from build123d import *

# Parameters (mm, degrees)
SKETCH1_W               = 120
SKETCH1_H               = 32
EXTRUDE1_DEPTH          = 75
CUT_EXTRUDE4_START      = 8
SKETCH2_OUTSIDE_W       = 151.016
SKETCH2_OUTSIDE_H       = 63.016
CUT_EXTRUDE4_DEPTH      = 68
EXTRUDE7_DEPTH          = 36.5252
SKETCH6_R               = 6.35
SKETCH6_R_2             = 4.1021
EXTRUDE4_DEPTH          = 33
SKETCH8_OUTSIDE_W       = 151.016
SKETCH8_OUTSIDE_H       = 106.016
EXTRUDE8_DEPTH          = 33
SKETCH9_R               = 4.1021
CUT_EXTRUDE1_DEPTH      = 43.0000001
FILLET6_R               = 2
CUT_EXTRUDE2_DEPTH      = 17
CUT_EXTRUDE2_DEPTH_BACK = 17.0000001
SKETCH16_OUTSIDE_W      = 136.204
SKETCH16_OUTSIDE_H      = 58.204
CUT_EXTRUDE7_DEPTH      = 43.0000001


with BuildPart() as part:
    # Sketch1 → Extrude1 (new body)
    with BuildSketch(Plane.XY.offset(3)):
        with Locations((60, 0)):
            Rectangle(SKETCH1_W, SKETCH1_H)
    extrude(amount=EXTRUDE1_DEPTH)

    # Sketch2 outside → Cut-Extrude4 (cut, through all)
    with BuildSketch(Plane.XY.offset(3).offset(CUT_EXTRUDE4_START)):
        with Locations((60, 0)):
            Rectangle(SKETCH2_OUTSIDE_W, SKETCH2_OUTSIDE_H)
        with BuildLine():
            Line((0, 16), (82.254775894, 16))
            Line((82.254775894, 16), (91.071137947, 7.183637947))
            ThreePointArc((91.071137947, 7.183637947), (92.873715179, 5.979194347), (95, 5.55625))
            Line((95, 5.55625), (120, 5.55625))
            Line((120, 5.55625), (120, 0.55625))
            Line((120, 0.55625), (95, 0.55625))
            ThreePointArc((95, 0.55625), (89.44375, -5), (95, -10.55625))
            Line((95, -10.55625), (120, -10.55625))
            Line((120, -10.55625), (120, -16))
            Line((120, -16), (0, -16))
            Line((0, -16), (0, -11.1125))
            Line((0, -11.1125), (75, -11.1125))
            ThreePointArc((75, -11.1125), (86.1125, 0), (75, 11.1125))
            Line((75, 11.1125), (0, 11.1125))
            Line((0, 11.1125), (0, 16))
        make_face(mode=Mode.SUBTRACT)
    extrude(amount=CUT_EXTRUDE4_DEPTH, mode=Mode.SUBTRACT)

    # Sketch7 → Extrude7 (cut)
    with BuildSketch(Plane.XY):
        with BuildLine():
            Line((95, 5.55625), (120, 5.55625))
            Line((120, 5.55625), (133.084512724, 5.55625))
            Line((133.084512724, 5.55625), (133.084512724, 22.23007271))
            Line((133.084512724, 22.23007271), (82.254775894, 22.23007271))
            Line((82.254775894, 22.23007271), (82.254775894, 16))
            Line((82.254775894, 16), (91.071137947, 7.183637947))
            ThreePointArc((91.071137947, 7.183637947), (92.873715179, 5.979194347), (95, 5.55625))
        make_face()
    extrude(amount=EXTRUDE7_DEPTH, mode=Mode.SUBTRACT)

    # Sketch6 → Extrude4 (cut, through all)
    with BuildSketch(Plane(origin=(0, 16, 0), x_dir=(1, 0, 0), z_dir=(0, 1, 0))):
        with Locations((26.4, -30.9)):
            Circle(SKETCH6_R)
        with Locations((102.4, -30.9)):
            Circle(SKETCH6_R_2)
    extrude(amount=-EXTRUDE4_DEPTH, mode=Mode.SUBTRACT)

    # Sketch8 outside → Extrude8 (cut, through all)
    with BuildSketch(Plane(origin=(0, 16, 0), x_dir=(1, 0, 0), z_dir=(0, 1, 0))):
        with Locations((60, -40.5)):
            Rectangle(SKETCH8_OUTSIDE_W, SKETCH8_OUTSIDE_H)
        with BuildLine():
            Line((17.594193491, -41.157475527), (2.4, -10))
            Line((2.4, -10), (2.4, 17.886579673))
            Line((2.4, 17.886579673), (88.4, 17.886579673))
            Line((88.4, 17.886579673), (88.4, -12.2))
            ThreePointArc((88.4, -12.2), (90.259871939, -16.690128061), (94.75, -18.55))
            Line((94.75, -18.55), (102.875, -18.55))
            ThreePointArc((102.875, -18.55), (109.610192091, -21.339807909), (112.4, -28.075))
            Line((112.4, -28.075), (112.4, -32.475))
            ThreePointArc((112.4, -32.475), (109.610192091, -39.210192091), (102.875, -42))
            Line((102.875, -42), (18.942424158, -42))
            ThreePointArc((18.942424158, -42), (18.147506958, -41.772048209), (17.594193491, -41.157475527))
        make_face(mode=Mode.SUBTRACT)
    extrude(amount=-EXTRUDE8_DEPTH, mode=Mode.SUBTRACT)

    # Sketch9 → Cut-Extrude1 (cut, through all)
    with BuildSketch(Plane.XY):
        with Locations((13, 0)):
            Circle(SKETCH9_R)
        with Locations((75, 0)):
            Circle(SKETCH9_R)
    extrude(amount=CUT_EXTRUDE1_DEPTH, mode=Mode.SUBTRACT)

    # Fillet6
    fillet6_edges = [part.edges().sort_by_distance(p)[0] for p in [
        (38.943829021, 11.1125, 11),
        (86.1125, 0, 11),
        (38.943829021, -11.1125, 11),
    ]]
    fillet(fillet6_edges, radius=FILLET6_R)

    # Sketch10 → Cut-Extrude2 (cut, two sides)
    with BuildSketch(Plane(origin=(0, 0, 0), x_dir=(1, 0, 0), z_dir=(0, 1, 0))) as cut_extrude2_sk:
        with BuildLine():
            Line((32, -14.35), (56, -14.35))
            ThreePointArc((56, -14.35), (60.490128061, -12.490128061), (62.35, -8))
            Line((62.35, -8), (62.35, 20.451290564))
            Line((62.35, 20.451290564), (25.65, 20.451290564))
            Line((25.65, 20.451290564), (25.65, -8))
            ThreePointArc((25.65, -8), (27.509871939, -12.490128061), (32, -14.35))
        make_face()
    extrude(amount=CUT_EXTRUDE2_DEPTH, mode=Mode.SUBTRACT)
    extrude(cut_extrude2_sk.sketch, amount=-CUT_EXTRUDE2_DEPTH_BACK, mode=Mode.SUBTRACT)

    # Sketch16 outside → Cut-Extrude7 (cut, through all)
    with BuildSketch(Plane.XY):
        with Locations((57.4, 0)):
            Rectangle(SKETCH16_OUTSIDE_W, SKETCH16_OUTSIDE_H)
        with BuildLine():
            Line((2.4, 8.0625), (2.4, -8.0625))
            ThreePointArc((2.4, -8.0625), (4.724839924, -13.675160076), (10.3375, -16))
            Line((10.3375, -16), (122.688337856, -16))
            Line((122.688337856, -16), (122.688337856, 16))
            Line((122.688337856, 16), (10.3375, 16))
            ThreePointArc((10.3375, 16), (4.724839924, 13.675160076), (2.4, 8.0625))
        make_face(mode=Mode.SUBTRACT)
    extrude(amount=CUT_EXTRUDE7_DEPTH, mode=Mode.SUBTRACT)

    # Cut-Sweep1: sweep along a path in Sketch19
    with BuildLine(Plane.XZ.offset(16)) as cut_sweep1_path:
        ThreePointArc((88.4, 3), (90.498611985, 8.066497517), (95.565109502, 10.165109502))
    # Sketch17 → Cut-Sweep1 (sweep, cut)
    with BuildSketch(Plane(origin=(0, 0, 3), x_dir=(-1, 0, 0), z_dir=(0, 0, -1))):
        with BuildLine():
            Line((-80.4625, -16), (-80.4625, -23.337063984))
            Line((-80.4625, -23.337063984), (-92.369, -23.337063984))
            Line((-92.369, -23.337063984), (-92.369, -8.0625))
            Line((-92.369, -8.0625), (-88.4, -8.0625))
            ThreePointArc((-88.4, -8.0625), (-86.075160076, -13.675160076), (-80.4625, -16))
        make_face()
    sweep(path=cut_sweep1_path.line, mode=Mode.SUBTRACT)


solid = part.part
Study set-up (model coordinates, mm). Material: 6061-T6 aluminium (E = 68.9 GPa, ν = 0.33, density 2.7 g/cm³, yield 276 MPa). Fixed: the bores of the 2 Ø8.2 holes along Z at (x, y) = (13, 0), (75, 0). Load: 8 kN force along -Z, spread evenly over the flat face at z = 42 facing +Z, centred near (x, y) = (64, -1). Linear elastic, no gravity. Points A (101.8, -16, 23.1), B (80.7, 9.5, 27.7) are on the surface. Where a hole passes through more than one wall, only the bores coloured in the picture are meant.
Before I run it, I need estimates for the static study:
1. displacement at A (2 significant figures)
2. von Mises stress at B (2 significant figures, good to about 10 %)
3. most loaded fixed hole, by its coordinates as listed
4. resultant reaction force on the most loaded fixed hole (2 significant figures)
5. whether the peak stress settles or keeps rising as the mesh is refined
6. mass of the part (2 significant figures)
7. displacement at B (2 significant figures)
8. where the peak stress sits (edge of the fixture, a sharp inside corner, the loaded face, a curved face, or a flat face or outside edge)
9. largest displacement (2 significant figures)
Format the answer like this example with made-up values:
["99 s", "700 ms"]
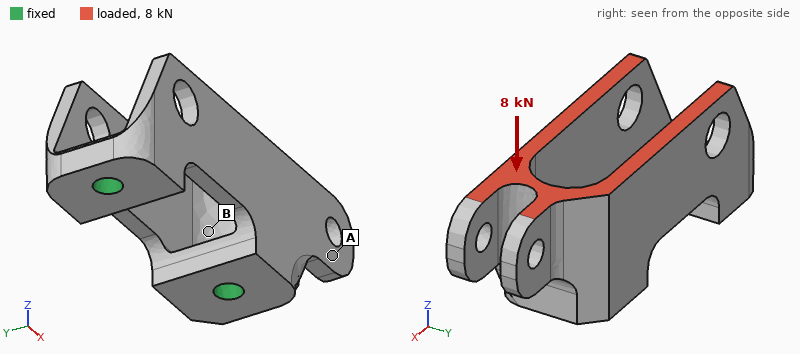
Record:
["33 µm", "17 MPa", "(75, 0)", "6.3 kN", "keeps rising", "110 g", "17 µm", "edge of the fixture", "42 µm"]
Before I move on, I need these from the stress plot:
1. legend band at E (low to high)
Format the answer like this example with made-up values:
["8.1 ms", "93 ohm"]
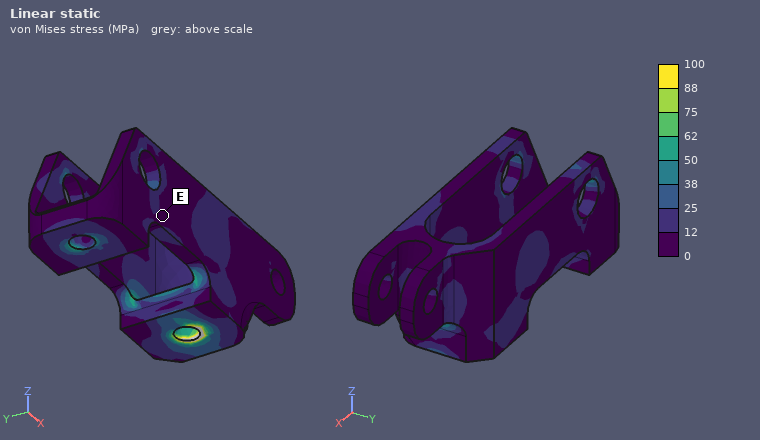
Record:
["0 to 12 MPa"]
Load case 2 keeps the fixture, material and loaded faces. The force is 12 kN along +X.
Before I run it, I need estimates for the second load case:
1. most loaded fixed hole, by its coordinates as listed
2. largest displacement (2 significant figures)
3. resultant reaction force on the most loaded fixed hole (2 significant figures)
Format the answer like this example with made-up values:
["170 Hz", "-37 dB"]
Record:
["(13, 0)", "0.17 mm", "8.7 kN"]
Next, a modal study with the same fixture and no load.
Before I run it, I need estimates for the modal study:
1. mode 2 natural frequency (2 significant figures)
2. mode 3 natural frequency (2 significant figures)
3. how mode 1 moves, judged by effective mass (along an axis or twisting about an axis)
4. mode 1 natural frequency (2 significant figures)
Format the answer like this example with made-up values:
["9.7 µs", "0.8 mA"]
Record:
["3500 Hz", "4800 Hz", "along Y", "3200 Hz"]
